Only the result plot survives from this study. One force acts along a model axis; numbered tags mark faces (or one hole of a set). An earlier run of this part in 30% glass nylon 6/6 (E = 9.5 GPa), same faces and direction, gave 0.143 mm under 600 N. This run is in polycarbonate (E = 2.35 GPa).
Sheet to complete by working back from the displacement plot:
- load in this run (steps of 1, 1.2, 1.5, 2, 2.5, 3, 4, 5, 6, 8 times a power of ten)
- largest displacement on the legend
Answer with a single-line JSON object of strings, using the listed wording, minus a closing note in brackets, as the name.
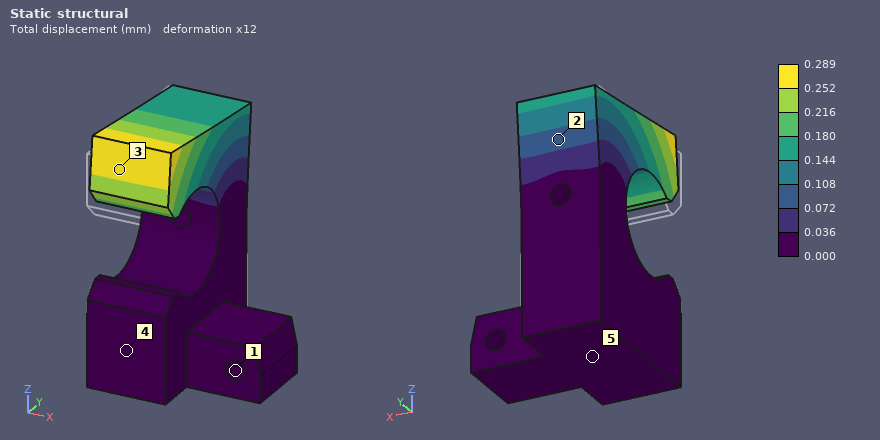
{"load in this run": "300 N", "largest displacement on the legend": "0.289 mm"}
